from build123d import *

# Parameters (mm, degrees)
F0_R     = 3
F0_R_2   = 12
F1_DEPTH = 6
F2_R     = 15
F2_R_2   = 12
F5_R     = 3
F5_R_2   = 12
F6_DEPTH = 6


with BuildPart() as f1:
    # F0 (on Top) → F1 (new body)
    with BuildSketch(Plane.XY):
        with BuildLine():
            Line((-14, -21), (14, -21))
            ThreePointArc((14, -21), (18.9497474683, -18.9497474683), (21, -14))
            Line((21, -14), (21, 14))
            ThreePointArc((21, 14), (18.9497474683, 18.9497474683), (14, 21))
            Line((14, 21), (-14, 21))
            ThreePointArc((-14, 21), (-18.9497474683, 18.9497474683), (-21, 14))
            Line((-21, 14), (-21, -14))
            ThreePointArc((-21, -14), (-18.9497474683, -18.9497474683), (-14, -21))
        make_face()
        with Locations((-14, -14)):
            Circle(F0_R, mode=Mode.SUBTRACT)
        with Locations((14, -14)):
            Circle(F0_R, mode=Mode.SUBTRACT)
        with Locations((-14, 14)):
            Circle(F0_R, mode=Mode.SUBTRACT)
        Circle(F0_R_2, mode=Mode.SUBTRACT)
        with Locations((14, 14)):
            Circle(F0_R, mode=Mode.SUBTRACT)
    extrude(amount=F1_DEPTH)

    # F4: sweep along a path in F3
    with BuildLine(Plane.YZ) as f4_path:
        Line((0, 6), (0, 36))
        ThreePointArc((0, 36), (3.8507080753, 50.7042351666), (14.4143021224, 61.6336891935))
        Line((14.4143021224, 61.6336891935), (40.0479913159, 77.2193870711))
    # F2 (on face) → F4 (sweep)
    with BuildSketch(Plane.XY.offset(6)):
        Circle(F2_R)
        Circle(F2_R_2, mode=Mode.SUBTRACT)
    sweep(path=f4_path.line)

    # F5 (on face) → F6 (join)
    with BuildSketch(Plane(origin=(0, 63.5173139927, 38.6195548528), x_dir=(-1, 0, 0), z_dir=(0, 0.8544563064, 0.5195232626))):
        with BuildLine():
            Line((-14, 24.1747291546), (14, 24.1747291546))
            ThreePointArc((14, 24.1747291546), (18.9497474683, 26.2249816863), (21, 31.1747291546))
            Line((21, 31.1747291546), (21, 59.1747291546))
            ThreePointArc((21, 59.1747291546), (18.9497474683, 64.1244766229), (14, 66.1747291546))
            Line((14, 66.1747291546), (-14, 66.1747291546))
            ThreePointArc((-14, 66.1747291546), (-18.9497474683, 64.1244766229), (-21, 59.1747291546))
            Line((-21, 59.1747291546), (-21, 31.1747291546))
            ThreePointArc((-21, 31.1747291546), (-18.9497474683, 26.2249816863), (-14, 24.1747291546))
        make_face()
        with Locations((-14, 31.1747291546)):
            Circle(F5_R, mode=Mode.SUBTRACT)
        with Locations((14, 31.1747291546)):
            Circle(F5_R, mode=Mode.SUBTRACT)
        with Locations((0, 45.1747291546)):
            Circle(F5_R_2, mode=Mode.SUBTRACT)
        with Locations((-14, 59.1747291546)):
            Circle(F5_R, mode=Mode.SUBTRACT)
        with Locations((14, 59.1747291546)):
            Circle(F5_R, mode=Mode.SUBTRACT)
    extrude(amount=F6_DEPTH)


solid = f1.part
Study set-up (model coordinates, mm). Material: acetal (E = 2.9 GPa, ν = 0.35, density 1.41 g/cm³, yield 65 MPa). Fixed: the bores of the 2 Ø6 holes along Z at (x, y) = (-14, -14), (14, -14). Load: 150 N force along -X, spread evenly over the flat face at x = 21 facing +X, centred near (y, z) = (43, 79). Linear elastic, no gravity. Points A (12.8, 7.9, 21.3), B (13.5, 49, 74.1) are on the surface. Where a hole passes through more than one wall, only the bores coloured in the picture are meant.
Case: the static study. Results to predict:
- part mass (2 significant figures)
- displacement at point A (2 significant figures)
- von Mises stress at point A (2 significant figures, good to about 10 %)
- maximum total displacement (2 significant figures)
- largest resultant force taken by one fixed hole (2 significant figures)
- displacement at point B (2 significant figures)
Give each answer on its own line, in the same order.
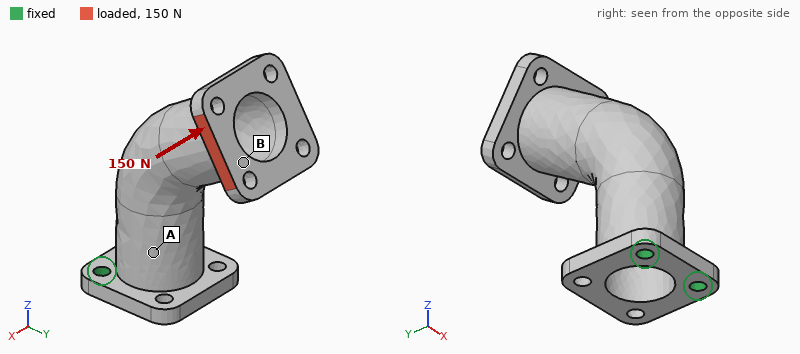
52 g
0.25 mm
5.1 MPa
1.5 mm
520 N
1.4 mm
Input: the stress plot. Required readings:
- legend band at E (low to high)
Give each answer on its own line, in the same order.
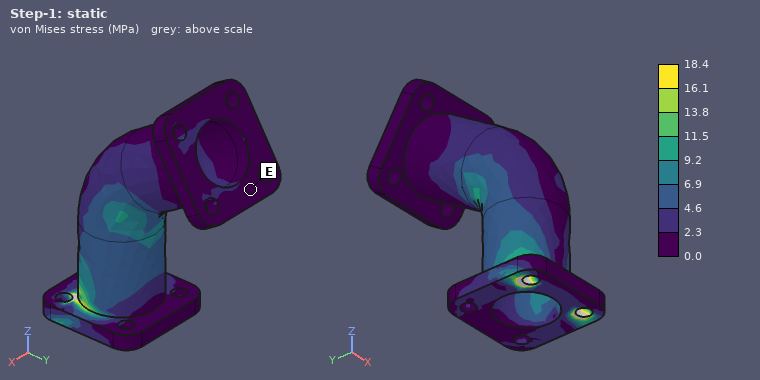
0.0 to 2.3 MPa
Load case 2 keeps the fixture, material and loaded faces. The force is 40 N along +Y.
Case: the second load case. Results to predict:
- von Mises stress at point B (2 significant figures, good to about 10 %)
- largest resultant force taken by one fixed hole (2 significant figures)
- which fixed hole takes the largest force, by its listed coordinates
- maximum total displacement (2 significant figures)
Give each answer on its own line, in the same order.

1.6 MPa
47 N
(14, -14)
1.4 mm
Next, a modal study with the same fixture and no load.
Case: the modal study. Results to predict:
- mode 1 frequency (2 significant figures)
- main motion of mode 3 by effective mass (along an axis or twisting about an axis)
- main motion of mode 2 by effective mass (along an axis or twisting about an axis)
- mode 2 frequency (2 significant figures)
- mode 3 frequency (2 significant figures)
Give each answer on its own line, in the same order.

180 Hz
twisting about Z
along X
390 Hz
1200 Hz
